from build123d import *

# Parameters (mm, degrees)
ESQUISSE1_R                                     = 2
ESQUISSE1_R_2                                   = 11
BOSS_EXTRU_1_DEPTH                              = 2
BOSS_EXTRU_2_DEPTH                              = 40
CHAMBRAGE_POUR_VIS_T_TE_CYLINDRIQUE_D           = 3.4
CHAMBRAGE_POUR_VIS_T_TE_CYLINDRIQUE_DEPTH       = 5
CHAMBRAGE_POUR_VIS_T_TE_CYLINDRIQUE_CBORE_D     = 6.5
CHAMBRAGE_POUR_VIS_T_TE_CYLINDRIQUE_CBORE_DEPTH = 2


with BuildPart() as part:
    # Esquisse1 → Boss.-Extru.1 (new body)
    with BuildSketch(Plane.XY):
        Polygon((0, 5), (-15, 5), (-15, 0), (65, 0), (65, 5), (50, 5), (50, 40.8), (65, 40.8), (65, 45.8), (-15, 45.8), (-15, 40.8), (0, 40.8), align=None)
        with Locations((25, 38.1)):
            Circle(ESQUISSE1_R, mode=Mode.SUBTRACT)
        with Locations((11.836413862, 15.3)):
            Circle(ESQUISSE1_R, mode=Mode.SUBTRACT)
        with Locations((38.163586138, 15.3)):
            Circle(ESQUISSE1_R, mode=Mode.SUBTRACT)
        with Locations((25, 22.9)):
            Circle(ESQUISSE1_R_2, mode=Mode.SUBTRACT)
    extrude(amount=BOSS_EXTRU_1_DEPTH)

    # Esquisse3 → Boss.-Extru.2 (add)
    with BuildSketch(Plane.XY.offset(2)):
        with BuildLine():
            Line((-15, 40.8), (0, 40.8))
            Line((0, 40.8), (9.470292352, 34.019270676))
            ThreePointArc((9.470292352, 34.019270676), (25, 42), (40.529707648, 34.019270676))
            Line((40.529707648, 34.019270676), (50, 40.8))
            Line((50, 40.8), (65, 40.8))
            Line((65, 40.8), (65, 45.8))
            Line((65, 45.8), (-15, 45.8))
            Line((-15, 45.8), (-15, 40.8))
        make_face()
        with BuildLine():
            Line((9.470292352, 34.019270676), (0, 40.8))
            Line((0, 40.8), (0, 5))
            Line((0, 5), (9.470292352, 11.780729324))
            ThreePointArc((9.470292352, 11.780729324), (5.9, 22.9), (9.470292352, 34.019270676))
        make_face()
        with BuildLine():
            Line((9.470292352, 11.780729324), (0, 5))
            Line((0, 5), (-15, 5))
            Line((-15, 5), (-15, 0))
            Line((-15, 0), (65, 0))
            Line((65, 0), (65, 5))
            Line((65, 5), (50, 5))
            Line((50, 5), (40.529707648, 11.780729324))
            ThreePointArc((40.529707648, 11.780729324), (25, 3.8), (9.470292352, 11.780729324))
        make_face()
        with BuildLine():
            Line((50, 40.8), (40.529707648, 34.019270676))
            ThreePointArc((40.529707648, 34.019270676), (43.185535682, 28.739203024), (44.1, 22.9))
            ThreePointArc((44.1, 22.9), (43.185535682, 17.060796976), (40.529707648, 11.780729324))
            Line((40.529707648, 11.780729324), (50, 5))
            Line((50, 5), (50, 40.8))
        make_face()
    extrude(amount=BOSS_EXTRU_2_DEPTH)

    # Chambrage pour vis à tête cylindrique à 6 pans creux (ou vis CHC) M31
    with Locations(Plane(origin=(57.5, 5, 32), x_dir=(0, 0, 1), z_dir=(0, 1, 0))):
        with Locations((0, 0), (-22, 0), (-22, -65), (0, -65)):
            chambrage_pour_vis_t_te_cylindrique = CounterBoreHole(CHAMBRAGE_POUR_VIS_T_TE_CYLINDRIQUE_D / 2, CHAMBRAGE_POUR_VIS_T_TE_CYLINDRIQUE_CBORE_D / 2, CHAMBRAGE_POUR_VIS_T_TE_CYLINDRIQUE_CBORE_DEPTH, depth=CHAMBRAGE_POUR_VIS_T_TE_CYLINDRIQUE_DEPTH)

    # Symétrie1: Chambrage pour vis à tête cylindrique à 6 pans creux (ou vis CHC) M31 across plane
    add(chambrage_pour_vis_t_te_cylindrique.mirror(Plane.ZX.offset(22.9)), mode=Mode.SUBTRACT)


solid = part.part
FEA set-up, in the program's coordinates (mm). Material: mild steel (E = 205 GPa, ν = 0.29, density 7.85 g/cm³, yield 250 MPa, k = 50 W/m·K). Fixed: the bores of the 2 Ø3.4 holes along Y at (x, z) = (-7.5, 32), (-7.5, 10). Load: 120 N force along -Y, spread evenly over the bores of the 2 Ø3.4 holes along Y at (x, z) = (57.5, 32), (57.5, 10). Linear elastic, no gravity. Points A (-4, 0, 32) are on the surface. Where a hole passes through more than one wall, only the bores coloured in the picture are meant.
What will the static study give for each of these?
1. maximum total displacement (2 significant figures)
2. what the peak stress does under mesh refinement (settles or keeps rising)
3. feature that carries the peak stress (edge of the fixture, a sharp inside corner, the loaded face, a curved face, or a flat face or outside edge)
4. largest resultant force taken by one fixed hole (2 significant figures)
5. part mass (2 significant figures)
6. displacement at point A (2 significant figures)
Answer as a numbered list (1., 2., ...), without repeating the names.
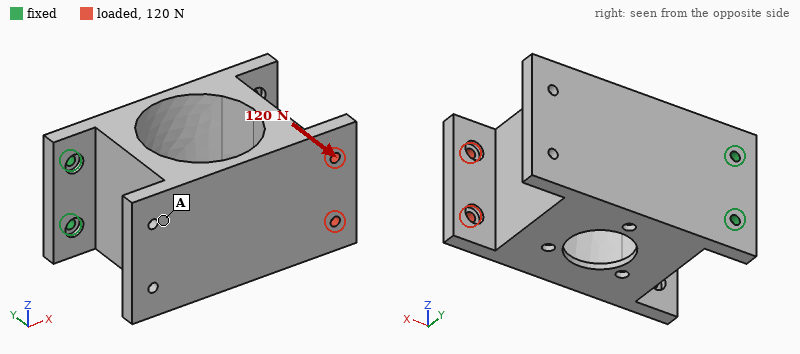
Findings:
1. 0.12 mm
2. keeps rising
3. edge of the fixture
4. 61 N
5. 480 g
6. 0.066 mm
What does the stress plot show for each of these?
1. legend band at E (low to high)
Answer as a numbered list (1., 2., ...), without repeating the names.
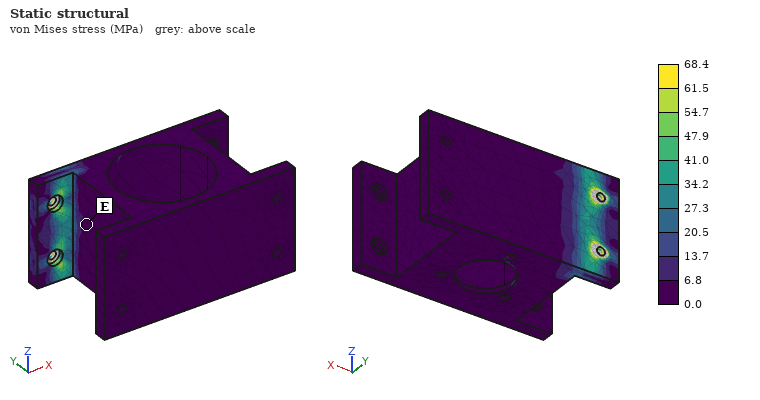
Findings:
1. 0.0 to 6.8 MPa
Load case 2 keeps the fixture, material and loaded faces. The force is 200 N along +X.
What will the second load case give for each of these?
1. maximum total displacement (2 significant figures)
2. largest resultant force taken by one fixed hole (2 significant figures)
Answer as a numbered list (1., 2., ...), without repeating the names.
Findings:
1. 0.14 mm
2. 100 N
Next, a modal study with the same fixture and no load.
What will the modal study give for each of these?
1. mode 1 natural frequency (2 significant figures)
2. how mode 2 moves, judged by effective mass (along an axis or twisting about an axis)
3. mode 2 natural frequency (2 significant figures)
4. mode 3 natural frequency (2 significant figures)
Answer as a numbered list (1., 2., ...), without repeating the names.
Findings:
1. 350 Hz
2. along Z
3. 1600 Hz
4. 2700 Hz
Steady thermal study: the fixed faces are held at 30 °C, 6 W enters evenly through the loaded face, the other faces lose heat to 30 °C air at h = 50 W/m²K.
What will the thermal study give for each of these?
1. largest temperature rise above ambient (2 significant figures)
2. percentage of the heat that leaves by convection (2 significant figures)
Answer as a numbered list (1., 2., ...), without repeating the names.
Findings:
1. 17 K
2. 82 %
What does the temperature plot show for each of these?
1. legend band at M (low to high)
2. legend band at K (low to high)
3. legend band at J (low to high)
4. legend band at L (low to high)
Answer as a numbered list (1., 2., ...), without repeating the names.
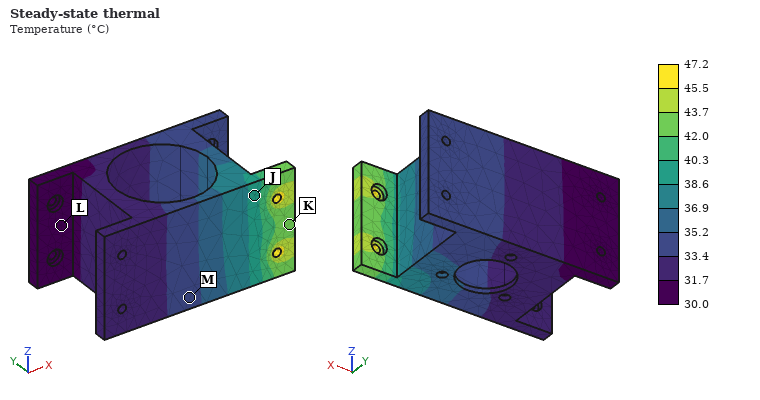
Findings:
1. 33.4 to 35.2 °C
2. 42.0 to 43.7 °C
3. 38.6 to 40.3 °C
4. 30.0 to 31.7 °C
